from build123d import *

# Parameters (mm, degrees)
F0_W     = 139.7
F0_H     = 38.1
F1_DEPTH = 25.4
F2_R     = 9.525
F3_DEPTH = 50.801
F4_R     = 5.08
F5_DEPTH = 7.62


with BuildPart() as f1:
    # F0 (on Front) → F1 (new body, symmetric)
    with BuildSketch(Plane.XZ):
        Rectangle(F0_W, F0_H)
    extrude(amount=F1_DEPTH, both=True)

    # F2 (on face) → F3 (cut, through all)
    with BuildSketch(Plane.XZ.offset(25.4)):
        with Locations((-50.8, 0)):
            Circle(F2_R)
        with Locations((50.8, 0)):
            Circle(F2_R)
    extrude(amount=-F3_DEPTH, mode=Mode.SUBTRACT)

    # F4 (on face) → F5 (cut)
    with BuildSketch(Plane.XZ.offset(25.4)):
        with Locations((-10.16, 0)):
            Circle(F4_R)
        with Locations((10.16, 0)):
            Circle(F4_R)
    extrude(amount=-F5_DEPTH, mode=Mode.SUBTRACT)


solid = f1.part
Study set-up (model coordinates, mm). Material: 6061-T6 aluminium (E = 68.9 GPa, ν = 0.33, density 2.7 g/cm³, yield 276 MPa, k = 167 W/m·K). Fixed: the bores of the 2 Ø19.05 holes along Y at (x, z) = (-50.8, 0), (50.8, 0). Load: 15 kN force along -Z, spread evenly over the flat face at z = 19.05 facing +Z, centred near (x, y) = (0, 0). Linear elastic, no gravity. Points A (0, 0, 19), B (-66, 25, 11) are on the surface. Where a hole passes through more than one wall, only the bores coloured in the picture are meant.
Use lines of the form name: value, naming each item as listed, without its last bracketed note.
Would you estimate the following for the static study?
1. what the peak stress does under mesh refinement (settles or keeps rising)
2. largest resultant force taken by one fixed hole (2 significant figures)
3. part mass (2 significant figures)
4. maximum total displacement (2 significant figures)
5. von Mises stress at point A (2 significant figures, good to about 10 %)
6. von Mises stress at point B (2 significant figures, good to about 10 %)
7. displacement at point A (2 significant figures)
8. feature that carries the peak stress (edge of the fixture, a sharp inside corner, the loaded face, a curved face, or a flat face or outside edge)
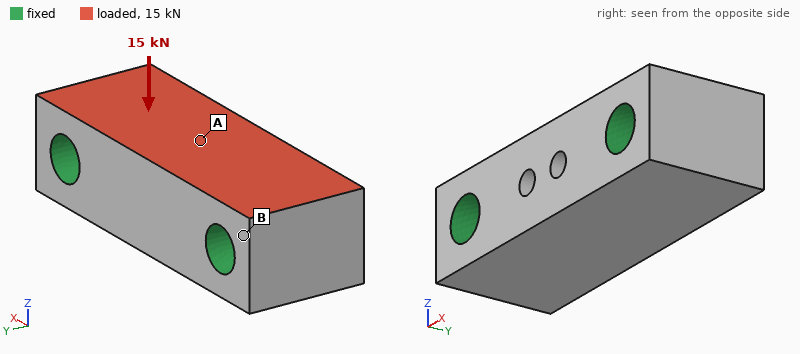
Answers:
what the peak stress does under mesh refinement: keeps rising
largest resultant force taken by one fixed hole: 7.5 kN
part mass: 650 g
maximum total displacement: 5.0 µm
von Mises stress at point A: 4.4 MPa
von Mises stress at point B: 1.7 MPa
displacement at point A: 4.4 µm
feature that carries the peak stress: edge of the fixture
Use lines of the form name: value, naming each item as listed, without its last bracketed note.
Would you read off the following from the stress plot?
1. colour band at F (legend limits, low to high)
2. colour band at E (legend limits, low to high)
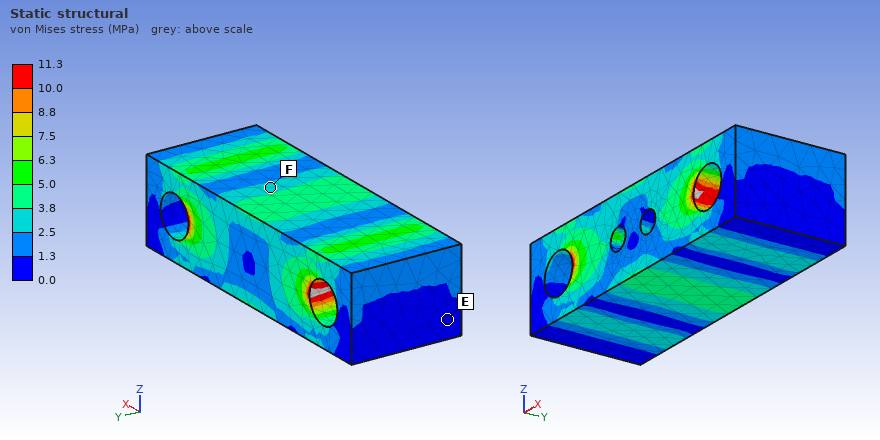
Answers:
colour band at F: 2.5 to 3.8 MPa
colour band at E: 0.0 to 1.3 MPa
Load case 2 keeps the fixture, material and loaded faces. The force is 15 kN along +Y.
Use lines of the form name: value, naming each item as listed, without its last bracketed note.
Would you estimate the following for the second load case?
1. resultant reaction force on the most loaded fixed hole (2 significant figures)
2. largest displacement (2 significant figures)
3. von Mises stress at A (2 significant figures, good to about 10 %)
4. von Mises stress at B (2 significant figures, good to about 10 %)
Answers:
resultant reaction force on the most loaded fixed hole: 7.5 kN
largest displacement: 9.0 µm
von Mises stress at A: 3.7 MPa
von Mises stress at B: 3.1 MPa
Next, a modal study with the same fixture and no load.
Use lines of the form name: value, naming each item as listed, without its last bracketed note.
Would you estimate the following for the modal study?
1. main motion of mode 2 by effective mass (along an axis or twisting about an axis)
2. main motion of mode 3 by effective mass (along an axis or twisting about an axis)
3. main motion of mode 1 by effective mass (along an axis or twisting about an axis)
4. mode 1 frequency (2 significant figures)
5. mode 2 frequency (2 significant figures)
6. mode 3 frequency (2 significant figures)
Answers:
main motion of mode 2 by effective mass: along Y
main motion of mode 3 by effective mass: twisting about X
main motion of mode 1 by effective mass: along Z
mode 1 frequency: 12 kHz
mode 2 frequency: 14 kHz
mode 3 frequency: 16 kHz
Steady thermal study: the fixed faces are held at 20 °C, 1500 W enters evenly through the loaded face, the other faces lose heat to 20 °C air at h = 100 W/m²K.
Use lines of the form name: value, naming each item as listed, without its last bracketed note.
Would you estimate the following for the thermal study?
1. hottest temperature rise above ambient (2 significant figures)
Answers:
hottest temperature rise above ambient: 51 K
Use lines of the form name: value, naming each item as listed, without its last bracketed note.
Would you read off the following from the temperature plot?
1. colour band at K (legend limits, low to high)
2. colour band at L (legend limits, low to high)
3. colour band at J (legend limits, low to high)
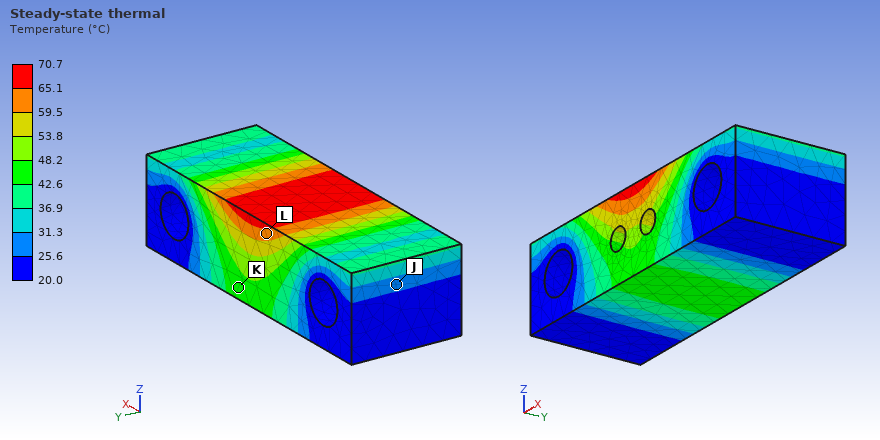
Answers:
colour band at K: 42.6 to 48.2 °C
colour band at L: 59.5 to 65.1 °C
colour band at J: 25.6 to 31.3 °C
